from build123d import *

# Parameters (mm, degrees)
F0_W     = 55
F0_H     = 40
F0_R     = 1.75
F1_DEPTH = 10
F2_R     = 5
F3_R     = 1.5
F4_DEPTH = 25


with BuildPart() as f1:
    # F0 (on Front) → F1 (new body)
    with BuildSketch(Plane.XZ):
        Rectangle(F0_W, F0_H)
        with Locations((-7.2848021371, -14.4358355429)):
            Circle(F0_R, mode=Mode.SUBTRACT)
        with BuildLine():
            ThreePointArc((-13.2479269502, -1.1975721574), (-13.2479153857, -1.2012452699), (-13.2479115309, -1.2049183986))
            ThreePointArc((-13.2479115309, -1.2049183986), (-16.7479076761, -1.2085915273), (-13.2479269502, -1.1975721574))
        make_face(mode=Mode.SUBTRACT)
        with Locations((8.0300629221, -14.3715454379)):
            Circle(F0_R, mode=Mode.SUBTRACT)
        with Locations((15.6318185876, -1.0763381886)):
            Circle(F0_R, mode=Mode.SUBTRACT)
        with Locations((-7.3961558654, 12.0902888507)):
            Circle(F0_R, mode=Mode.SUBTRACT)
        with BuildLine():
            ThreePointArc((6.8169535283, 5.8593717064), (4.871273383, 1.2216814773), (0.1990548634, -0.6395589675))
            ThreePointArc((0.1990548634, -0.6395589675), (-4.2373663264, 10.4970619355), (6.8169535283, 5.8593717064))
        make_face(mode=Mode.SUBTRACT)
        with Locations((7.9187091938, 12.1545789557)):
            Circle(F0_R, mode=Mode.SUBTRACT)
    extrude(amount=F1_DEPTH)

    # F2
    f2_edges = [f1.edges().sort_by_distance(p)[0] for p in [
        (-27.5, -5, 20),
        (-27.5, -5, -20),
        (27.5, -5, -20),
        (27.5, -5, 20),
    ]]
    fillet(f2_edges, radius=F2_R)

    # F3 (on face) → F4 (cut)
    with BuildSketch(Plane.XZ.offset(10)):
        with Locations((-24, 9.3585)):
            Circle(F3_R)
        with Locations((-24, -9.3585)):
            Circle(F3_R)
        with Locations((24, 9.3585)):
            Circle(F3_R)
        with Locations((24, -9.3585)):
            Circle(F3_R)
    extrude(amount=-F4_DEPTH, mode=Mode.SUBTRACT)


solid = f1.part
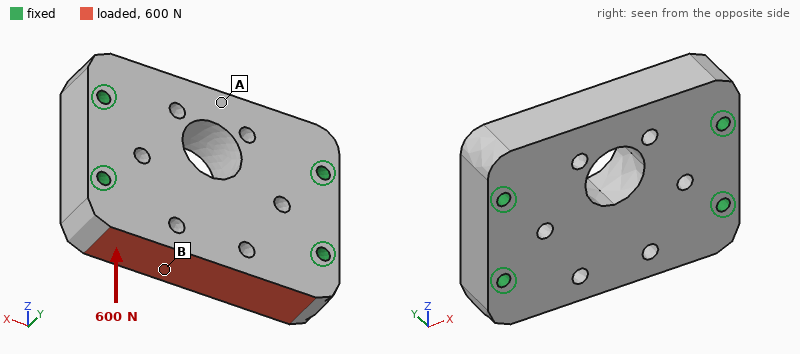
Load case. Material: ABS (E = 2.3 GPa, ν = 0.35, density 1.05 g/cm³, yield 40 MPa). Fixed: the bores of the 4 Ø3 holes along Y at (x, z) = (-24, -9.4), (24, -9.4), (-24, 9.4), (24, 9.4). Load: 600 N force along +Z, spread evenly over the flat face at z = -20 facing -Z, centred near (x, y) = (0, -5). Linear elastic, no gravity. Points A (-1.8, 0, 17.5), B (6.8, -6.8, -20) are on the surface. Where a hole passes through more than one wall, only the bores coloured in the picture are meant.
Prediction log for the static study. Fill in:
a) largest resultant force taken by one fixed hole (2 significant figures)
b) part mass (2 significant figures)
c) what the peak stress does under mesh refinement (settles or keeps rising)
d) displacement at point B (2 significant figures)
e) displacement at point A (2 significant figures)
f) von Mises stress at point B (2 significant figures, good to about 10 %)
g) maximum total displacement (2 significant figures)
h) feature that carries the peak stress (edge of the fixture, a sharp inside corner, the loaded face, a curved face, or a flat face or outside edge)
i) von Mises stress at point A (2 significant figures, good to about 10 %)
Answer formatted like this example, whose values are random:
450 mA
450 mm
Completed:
180 N
21 g
keeps rising
27 µm
13 µm
2.0 MPa
29 µm
edge of the fixture
0.74 MPa
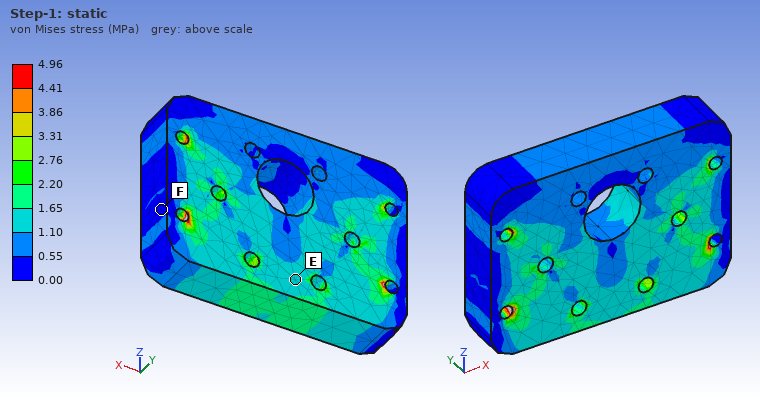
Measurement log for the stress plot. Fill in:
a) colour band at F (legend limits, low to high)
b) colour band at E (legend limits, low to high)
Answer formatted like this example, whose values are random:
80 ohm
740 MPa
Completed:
0.00 to 0.55 MPa
1.10 to 1.65 MPa
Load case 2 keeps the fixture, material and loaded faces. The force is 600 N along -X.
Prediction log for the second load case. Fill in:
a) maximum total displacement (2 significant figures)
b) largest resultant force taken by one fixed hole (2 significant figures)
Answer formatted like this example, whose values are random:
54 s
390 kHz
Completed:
26 µm
280 N
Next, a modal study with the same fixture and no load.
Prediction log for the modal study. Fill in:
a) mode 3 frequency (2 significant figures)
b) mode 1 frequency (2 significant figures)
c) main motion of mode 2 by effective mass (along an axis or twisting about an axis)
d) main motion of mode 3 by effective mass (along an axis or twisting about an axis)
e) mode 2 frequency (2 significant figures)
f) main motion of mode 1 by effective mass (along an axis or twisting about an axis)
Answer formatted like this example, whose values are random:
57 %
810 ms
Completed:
7500 Hz
4500 Hz
twisting about X
along Z
5200 Hz
along Y
